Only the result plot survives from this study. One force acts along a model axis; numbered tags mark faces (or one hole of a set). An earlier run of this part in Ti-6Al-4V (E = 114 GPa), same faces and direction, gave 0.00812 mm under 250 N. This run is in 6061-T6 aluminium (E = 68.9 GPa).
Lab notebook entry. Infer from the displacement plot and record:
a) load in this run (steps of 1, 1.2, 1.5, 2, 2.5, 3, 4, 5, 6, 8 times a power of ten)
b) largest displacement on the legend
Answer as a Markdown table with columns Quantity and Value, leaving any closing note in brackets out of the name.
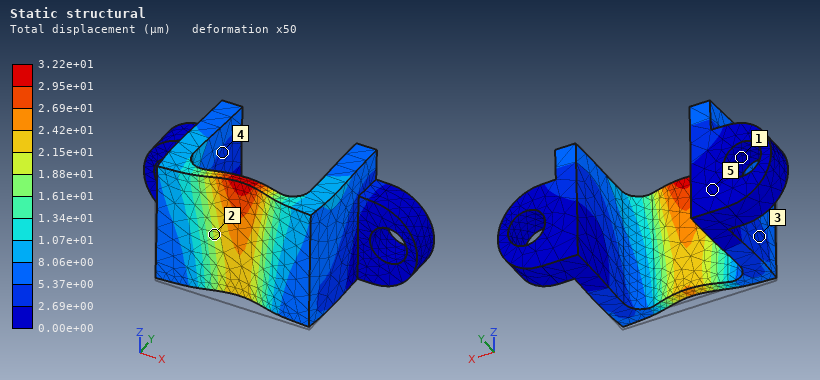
| Quantity | Value |
|---|---|
| load in this run | 600 N |
| largest displacement on the legend | 3.22e+01 µm |
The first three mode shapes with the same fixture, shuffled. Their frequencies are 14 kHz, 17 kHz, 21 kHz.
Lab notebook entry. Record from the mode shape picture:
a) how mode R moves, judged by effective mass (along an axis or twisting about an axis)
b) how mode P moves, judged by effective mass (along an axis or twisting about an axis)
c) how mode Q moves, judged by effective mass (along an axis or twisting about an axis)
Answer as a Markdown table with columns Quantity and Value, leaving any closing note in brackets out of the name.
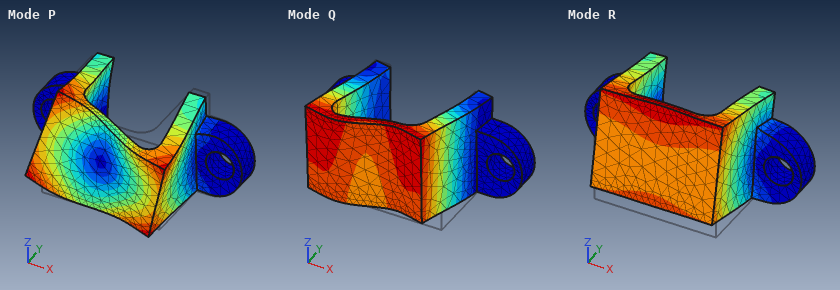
| Quantity | Value |
|---|---|
| how mode R moves, judged by effective mass | along Z |
| how mode P moves, judged by effective mass | twisting about Y |
| how mode Q moves, judged by effective mass | along X |
